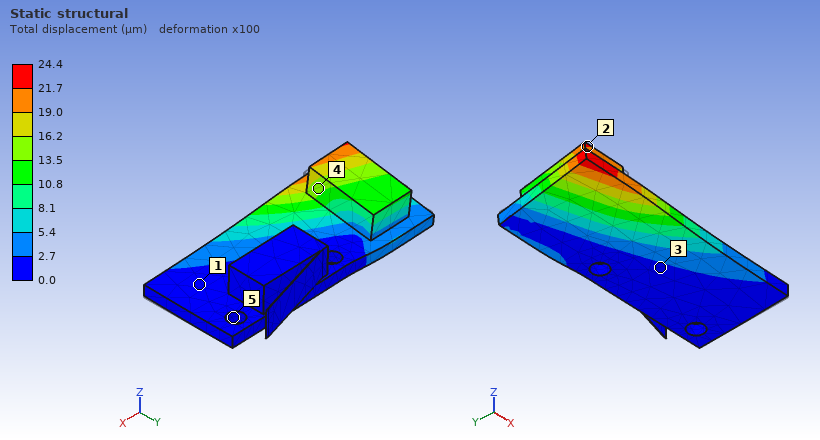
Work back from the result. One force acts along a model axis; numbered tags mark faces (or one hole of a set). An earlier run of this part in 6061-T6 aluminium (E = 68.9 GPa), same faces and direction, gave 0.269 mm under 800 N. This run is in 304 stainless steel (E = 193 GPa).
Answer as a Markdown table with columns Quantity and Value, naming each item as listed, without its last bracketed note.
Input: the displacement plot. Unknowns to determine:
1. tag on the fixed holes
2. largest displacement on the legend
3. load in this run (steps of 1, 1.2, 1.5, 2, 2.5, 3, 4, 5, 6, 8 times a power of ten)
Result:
| Quantity | Value |
|---|---|
| tag on the fixed holes | 5 |
| largest displacement on the legend | 24.4 µm |
| load in this run | 200 N |
